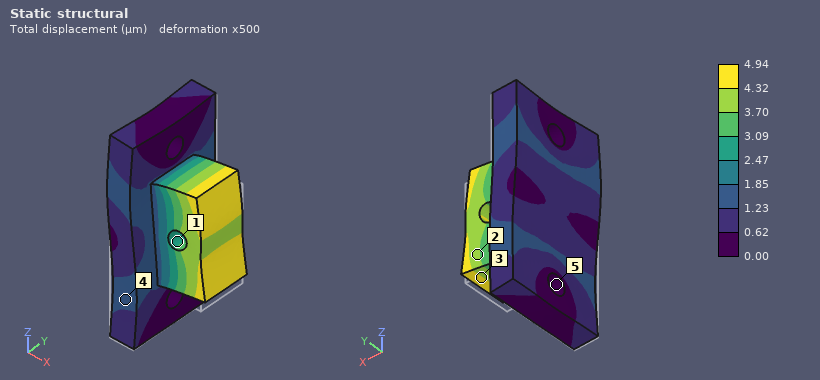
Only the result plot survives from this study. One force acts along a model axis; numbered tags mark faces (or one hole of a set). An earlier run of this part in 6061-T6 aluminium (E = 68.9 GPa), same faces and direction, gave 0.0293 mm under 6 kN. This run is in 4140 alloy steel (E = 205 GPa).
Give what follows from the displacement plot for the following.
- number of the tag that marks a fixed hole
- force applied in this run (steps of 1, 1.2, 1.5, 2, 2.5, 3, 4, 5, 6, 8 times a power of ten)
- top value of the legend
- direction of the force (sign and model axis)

5
3 kN
4.94 µm
+Z
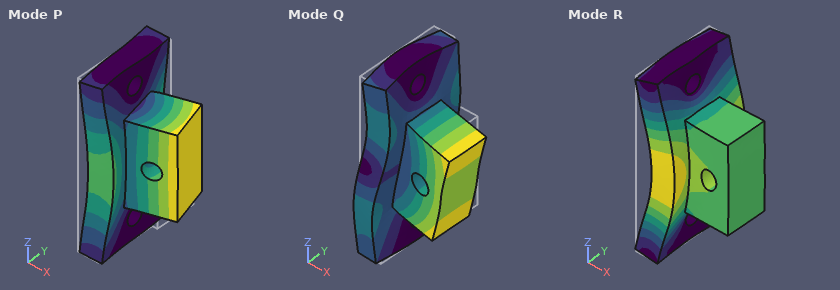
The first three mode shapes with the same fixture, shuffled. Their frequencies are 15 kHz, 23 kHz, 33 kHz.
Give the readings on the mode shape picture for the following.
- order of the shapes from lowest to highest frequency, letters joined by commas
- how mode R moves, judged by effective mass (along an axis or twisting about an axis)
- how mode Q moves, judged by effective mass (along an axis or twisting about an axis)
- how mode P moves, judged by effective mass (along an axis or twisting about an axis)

P, R, Q
along X
along Z
along Y
